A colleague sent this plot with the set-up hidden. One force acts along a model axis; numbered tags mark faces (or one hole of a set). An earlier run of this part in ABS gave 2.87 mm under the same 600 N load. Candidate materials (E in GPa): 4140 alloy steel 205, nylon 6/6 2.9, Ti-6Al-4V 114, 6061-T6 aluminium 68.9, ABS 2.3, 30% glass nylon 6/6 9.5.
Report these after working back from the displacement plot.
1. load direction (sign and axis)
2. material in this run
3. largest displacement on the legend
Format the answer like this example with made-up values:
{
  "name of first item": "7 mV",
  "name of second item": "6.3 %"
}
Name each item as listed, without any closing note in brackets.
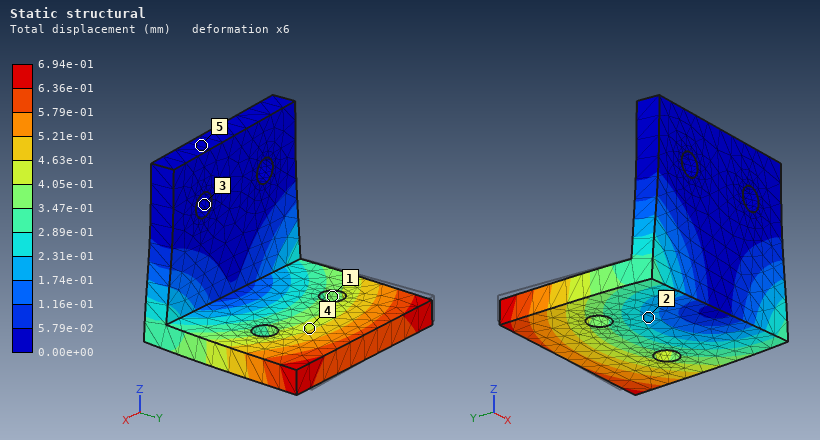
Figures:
{
  "load direction": "+X",
  "material in this run": "30% glass nylon 6/6",
  "largest displacement on the legend": "6.94e-01 mm"
}
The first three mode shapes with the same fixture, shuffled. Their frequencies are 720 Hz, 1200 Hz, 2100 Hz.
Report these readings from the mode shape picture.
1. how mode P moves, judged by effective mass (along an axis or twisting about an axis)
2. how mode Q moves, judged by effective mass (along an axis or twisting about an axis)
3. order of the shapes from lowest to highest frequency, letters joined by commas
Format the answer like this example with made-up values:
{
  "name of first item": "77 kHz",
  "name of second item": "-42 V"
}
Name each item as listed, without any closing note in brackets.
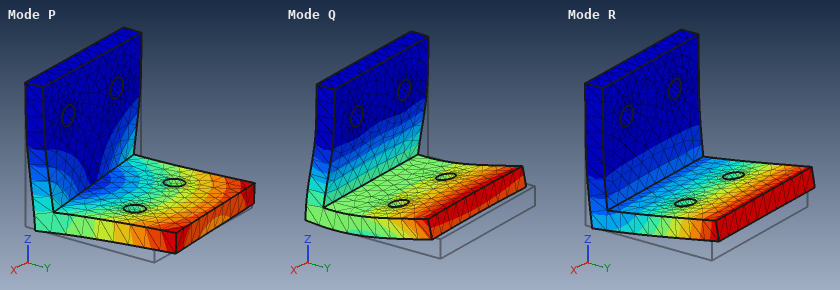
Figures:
{
  "how mode P moves, judged by effective mass": "along X",
  "how mode Q moves, judged by effective mass": "along Y",
  "order of the shapes from lowest to highest frequency, letters joined by commas": "R, P, Q"
}
